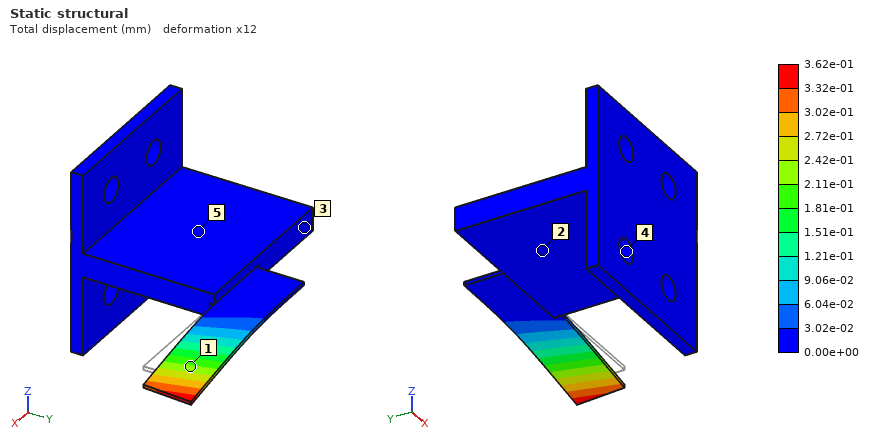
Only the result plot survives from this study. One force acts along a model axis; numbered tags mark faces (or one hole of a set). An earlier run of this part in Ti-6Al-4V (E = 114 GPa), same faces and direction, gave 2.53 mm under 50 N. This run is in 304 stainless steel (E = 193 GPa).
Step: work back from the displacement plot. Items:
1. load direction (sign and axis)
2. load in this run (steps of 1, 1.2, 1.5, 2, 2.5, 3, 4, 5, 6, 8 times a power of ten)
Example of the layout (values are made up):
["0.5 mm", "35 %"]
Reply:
["-Z", "12 N"]
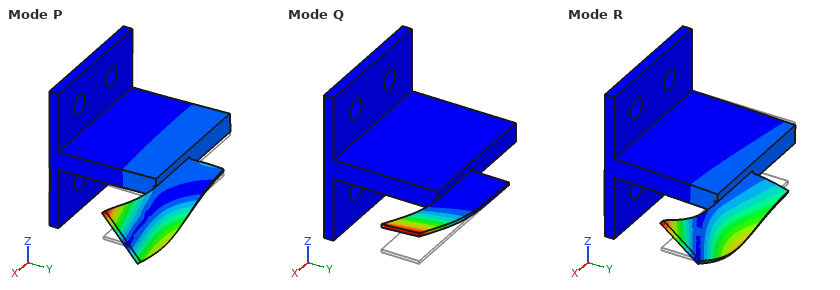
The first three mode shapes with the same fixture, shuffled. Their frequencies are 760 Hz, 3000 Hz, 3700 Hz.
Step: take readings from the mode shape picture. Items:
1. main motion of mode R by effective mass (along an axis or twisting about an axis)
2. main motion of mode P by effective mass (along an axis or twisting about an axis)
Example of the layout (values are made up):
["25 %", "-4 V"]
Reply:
["along Z", "along Z"]
